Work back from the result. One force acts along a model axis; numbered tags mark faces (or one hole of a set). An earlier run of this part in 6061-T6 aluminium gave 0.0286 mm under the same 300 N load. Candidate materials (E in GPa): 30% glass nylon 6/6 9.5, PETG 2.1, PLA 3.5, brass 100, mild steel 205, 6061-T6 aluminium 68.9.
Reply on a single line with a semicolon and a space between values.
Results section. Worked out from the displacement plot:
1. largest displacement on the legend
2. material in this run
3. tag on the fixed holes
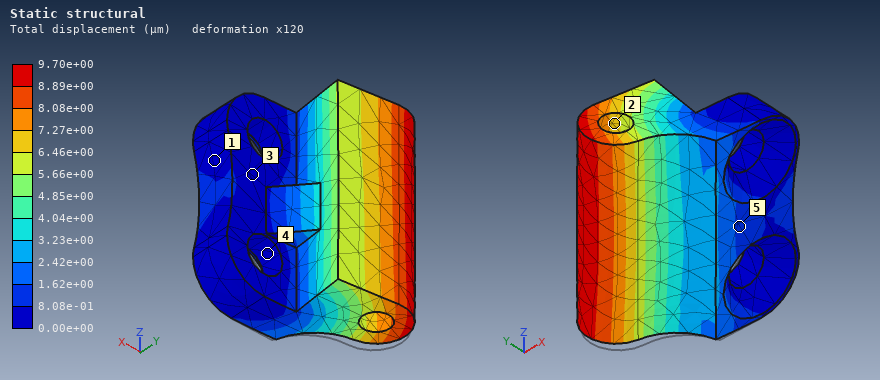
9.70e+00 µm; mild steel; 4
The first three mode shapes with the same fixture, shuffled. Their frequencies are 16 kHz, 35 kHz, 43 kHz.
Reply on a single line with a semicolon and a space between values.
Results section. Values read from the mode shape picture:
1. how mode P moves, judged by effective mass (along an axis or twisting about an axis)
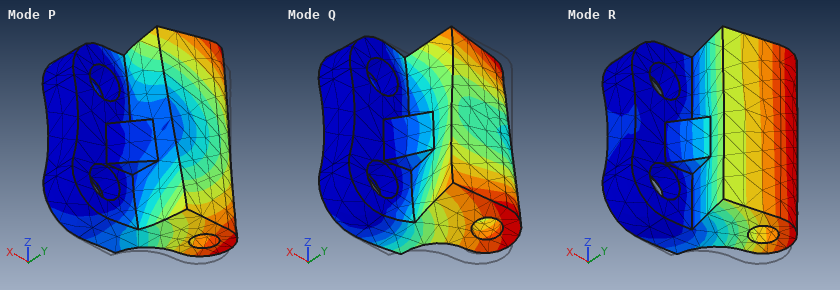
along Z
